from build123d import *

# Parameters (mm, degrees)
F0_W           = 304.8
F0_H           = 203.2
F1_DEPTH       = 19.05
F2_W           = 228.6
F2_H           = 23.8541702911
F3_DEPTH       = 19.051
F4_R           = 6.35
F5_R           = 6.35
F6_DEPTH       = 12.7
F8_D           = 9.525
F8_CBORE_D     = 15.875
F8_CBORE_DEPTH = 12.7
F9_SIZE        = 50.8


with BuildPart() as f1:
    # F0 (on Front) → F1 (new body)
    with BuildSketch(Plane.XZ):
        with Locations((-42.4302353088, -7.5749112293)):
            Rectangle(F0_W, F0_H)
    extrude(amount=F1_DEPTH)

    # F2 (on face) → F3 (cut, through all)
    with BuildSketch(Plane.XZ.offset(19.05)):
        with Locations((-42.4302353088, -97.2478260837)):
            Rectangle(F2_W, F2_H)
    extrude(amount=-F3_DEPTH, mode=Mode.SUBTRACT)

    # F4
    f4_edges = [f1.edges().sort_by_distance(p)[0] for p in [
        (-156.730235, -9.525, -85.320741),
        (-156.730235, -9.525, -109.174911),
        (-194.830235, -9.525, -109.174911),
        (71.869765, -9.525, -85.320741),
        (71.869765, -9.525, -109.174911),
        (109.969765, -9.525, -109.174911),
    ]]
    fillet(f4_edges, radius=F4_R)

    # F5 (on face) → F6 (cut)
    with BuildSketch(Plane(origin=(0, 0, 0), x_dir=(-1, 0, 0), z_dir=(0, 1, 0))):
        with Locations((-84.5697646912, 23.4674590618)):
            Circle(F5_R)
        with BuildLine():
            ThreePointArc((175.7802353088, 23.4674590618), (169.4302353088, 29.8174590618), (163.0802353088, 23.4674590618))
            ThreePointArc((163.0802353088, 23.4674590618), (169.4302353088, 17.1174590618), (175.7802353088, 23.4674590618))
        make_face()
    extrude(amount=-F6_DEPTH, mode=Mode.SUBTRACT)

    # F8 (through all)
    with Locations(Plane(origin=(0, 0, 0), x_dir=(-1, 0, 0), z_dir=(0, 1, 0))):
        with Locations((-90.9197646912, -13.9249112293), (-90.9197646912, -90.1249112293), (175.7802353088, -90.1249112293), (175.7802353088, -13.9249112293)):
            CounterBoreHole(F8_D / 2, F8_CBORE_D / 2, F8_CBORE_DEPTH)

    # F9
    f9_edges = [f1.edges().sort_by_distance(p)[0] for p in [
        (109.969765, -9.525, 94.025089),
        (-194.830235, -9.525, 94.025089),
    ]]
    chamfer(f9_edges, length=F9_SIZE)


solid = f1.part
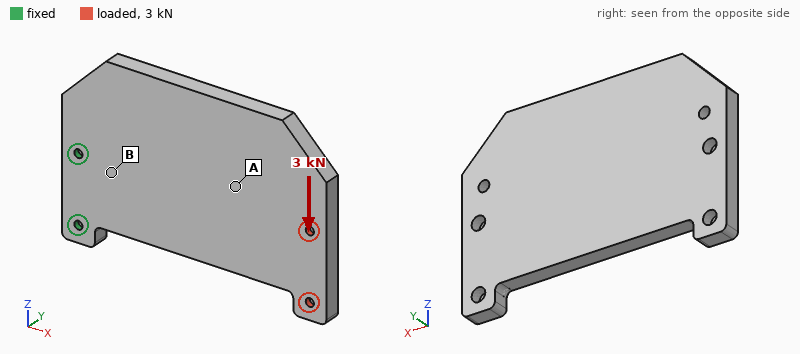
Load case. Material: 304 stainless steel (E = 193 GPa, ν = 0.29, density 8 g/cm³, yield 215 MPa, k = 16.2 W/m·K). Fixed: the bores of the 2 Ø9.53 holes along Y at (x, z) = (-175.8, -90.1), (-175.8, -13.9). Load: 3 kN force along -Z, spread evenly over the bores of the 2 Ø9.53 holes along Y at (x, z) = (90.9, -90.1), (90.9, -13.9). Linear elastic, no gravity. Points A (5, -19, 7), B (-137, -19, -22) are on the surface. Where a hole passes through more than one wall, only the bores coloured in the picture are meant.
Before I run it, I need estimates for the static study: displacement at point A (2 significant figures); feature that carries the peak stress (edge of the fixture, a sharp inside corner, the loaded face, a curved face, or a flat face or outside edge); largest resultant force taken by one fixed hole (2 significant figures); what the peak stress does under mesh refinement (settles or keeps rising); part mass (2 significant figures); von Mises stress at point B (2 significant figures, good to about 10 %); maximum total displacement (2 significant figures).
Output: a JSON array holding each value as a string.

["0.060 mm", "edge of the fixture", "10 kN", "keeps rising", "8.1 kg", "13 MPa", "0.10 mm"]
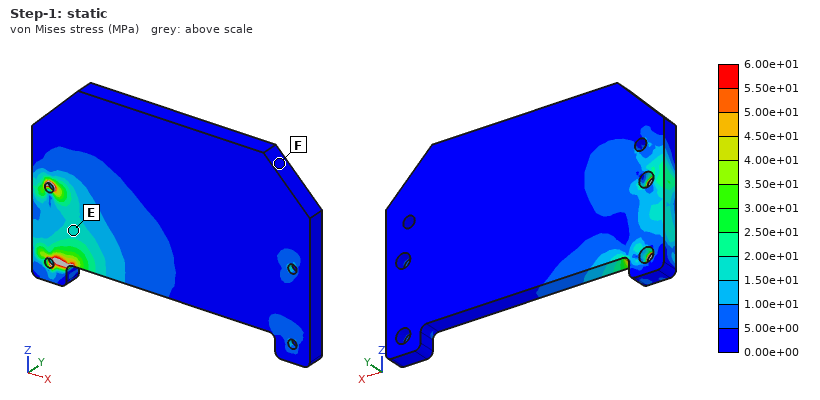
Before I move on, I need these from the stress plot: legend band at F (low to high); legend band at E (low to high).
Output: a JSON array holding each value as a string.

["0.00e+00 to 5.00e+00 MPa", "1.50e+01 to 2.00e+01 MPa"]
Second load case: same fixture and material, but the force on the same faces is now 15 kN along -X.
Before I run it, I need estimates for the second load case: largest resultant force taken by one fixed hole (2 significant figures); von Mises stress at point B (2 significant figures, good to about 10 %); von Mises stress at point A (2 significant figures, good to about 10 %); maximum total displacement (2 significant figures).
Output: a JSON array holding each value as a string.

["7.7 kN", "16 MPa", "12 MPa", "0.23 mm"]
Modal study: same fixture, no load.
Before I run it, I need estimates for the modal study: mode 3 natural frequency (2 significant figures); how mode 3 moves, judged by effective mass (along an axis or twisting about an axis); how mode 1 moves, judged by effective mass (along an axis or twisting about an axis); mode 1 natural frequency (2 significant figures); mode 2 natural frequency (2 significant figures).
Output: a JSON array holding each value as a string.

["590 Hz", "along Z", "along Y", "110 Hz", "450 Hz"]
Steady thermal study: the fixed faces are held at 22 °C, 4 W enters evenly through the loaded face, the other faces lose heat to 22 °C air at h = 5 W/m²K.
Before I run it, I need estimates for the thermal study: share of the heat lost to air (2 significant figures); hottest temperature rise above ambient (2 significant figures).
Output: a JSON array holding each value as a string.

["78 %", "18 K"]
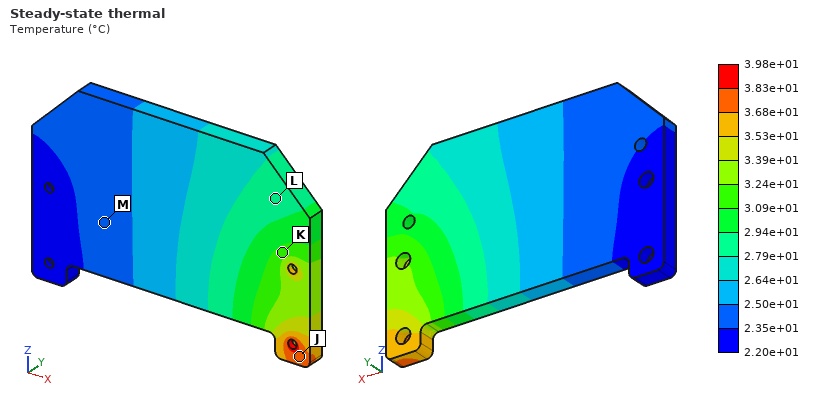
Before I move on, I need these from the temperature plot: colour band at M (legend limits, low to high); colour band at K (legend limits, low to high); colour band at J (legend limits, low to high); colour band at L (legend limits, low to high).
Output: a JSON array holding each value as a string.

["2.35e+01 to 2.50e+01 °C", "3.09e+01 to 3.24e+01 °C", "3.68e+01 to 3.83e+01 °C", "2.79e+01 to 2.94e+01 °C"]
